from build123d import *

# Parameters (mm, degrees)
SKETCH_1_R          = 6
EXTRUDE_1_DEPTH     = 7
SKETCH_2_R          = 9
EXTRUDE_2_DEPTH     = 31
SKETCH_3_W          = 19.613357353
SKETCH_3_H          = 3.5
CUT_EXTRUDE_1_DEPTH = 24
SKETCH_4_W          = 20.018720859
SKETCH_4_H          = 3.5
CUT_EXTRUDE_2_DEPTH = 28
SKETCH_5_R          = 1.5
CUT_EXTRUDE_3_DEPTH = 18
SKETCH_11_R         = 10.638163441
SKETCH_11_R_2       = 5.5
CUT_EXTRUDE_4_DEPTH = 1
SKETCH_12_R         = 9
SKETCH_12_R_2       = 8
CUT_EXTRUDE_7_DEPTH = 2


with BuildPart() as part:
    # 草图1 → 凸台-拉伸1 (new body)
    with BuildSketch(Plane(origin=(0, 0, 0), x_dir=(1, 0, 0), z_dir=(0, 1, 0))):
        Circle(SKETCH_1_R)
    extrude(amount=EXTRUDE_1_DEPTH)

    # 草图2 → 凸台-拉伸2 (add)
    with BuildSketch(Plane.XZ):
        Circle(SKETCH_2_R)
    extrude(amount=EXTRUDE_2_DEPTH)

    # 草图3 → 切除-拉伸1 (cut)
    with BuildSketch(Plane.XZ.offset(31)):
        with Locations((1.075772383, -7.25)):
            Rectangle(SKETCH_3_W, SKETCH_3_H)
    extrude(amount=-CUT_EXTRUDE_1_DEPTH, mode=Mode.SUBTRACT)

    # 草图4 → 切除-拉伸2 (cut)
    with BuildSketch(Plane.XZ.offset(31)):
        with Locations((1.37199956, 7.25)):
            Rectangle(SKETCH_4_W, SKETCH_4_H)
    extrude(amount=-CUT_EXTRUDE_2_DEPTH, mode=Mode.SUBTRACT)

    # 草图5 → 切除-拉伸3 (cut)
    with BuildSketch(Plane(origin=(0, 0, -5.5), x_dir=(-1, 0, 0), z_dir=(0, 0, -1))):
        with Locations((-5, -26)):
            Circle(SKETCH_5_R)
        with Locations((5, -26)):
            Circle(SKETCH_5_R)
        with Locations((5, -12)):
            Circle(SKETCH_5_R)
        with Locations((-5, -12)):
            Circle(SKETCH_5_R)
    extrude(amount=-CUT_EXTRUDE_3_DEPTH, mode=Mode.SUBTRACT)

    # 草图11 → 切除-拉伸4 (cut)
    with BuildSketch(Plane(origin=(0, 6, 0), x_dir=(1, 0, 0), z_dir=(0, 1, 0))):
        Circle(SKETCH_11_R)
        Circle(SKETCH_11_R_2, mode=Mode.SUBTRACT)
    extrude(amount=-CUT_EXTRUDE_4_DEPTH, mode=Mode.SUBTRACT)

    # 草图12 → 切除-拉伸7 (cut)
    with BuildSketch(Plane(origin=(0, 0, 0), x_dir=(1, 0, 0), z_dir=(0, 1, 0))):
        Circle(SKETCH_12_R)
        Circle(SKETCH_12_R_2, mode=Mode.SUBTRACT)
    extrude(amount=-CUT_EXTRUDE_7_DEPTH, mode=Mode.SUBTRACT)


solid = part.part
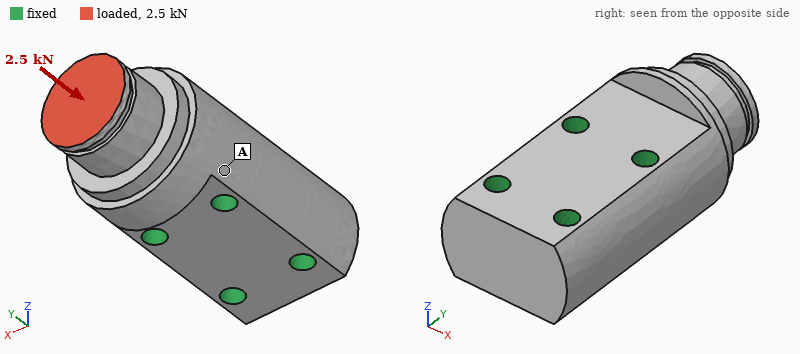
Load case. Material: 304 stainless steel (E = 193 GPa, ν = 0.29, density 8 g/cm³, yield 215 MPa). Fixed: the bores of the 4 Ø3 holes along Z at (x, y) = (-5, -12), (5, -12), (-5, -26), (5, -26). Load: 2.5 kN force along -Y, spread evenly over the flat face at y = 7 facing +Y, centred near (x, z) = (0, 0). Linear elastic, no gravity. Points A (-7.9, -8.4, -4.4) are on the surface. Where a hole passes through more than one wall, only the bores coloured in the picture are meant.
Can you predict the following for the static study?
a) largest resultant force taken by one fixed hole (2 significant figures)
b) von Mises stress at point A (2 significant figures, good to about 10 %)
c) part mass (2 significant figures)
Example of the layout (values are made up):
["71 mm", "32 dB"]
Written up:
["1.2 kN", "8.4 MPa", "51 g"]
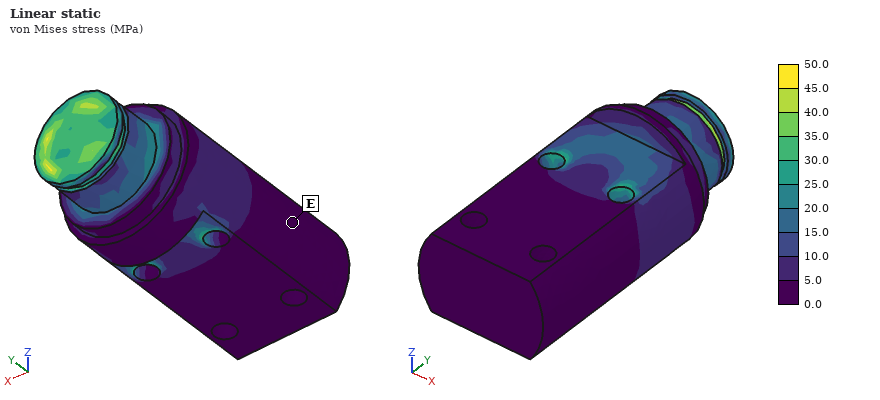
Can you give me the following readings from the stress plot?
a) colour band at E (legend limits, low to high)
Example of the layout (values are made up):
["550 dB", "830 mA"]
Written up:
["0.0 to 5.0 MPa"]
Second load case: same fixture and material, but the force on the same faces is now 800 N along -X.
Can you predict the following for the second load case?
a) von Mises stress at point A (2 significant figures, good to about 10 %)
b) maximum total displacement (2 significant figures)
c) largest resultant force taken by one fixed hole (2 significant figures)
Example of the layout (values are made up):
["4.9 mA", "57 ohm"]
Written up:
["19 MPa", "4.7 µm", "1.3 kN"]
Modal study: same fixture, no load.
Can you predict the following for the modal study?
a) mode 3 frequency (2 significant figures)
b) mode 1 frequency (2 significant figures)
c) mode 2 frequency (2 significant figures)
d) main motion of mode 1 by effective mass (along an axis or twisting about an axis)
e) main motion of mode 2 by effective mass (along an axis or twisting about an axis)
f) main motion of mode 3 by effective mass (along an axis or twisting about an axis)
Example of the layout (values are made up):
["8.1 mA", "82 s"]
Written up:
["49 kHz", "23 kHz", "31 kHz", "along Z", "along X", "twisting about Y"]
